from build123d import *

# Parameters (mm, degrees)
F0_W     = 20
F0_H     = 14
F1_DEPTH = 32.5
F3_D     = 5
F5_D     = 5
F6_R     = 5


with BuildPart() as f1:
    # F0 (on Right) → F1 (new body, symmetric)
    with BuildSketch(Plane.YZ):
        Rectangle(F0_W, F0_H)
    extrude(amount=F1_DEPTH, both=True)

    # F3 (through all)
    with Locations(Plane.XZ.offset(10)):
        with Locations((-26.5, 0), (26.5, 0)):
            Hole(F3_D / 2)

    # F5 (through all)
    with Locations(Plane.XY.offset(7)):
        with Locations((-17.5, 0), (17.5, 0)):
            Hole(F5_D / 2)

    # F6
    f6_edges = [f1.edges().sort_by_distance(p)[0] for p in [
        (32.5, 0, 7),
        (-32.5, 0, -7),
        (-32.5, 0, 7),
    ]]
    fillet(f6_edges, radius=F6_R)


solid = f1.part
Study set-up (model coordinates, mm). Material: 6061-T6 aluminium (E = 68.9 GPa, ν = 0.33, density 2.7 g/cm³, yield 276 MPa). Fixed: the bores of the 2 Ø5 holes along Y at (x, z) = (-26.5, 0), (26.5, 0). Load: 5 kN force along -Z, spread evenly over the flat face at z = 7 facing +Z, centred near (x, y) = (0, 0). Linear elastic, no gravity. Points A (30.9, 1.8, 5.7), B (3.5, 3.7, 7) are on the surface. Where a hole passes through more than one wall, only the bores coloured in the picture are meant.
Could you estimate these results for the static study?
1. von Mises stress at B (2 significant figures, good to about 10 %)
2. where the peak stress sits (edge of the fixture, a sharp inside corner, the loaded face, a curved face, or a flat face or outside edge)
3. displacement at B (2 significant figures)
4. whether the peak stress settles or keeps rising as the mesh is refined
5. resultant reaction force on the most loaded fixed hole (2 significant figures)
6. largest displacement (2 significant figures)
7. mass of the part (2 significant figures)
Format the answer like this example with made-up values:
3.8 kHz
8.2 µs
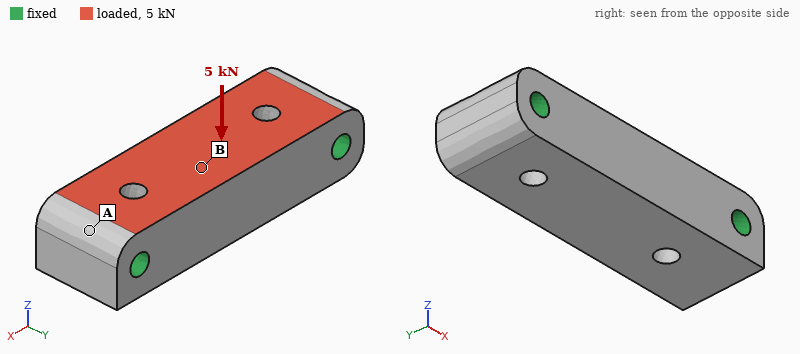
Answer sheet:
21 MPa
edge of the fixture
14 µm
keeps rising
2.5 kN
15 µm
45 g
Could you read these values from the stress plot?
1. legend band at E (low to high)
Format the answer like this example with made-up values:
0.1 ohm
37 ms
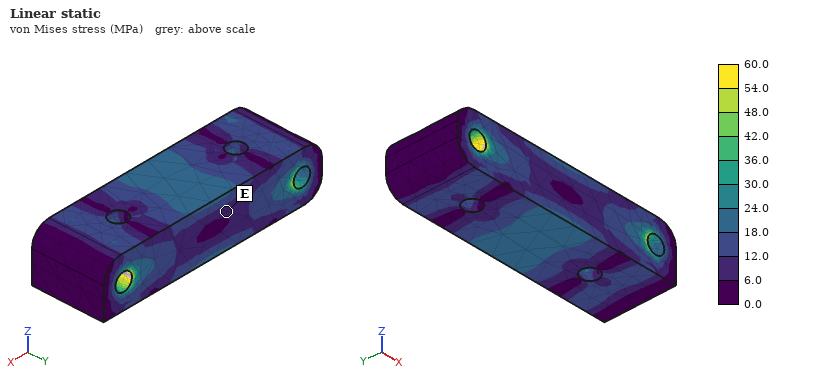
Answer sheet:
6.0 to 12.0 MPa
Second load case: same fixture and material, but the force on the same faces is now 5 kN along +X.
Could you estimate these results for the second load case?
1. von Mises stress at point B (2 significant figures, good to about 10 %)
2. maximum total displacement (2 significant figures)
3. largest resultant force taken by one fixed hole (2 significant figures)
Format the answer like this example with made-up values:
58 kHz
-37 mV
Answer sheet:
8.3 MPa
3.0 µm
2.6 kN
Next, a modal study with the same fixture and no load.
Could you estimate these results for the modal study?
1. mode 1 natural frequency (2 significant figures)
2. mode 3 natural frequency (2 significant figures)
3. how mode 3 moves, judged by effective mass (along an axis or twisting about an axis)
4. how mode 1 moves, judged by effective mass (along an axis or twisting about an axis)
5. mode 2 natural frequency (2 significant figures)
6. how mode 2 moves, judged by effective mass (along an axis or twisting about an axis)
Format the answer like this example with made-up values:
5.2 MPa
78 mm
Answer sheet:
16 kHz
25 kHz
twisting about X
along Z
21 kHz
along Y
